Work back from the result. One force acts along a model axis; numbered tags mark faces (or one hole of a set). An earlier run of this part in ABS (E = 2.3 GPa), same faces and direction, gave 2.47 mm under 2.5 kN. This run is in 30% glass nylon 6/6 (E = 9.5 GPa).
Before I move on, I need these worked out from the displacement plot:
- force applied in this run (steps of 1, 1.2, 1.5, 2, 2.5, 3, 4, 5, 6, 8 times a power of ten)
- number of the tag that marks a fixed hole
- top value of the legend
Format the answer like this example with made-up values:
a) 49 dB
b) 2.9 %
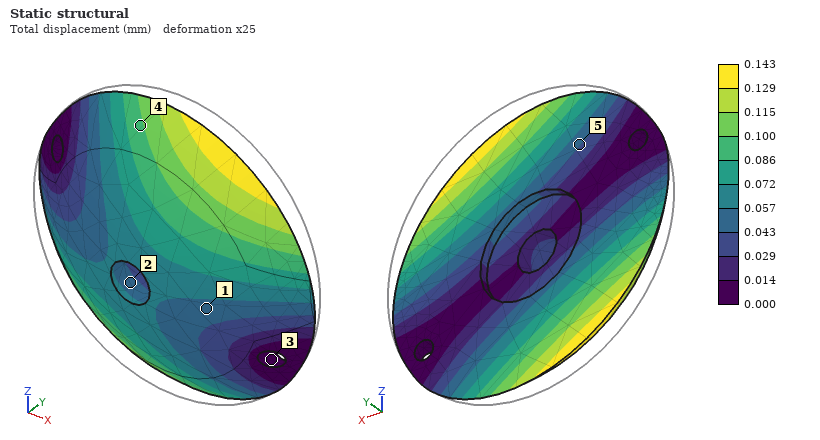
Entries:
a) 600 N
b) 3
c) 0.143 mm
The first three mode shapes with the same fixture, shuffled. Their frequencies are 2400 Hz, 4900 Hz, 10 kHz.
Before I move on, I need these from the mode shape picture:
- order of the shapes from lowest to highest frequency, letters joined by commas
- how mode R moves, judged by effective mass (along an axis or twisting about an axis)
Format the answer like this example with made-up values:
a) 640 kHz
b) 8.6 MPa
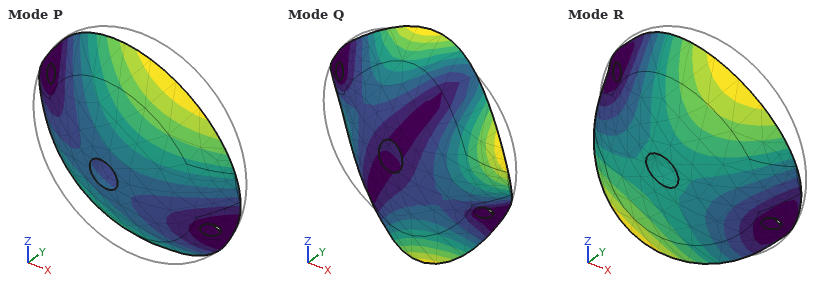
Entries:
a) P, R, Q
b) along Y
